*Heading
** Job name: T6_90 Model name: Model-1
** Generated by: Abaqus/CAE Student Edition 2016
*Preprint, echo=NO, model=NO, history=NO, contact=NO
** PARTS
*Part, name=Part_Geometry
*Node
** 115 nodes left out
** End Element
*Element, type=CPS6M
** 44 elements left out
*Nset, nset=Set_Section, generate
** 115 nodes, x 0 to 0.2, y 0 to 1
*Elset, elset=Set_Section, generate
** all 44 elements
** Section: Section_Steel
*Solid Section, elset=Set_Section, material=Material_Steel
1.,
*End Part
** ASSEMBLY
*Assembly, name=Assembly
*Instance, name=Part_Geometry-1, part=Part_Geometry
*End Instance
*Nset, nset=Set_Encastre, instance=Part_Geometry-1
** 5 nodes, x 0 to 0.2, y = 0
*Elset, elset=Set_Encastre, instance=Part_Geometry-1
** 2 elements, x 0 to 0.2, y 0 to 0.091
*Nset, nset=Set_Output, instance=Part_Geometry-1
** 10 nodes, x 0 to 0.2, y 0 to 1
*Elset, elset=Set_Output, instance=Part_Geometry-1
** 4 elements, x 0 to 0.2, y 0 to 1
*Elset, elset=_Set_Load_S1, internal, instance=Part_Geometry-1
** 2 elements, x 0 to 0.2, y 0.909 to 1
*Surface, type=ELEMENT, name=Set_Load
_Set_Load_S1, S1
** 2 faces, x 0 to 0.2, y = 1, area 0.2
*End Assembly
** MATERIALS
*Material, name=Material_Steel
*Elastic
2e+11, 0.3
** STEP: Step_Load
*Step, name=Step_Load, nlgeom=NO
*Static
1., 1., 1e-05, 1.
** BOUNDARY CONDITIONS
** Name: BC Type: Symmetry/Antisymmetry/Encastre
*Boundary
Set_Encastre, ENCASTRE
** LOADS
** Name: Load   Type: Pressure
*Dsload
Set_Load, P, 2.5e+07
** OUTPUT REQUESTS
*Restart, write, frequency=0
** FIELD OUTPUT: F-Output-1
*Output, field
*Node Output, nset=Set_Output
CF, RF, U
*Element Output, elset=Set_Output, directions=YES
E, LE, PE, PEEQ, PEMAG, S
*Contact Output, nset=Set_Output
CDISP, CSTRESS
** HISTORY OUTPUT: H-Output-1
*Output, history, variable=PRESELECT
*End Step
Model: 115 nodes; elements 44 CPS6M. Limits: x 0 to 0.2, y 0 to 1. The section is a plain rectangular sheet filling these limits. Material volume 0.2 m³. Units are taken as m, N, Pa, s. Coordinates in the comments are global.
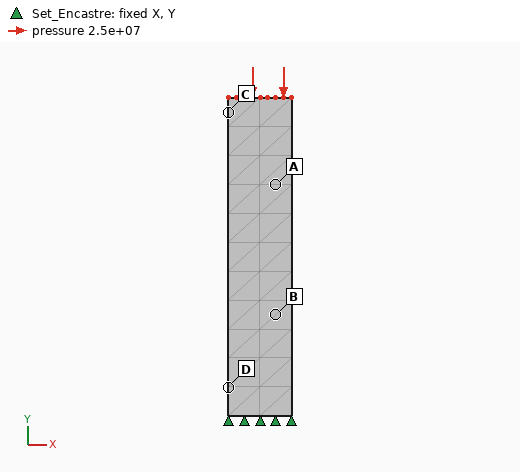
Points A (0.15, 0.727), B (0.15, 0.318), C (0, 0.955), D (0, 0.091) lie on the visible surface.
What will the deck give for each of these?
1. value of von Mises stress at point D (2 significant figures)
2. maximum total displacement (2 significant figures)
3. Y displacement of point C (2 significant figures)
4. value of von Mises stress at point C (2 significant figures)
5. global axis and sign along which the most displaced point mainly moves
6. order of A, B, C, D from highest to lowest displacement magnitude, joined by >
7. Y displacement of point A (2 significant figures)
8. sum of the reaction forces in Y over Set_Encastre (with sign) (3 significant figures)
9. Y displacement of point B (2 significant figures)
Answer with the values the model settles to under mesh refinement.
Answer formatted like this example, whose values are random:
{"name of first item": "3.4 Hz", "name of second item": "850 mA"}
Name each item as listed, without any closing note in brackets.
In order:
{"value of von Mises stress at point D": "2.4e+07 Pa", "maximum total displacement": "1.2e-04 m", "Y displacement of point C": "-1.2e-04 m", "value of von Mises stress at point C": "2.5e+07 Pa", "global axis and sign along which the most displaced point mainly moves": "-Y", "order of A, B, C, D from highest to lowest displacement magnitude, joined by >": "C > A > B > D", "Y displacement of point A": "-9.1e-05 m", "sum of the reaction forces in Y over Set_Encastre (with sign)": "5.00e+06 N", "Y displacement of point B": "-3.9e-05 m"}
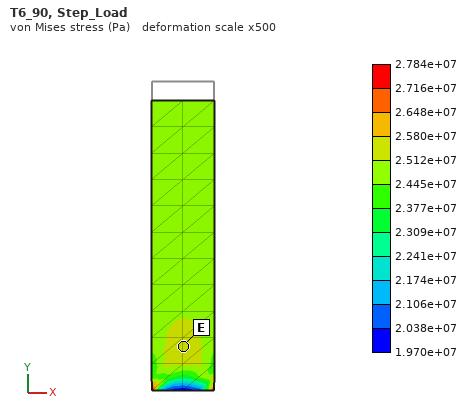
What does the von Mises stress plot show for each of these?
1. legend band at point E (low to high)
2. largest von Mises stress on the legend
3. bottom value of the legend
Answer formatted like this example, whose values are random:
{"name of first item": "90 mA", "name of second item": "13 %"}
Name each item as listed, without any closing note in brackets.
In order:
{"legend band at point E": "2.512e+07 to 2.580e+07 Pa", "largest von Mises stress on the legend": "2.784e+07 Pa", "bottom value of the legend": "1.970e+07 Pa"}
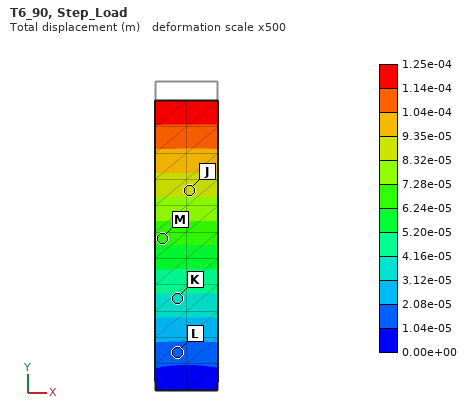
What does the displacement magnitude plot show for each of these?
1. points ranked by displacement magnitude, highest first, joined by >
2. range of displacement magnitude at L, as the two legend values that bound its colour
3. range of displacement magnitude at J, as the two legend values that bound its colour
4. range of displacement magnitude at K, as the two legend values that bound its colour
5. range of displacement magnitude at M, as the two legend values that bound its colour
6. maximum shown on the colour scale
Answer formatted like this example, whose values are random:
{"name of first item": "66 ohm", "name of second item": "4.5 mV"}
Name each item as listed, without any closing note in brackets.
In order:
{"points ranked by displacement magnitude, highest first, joined by >": "J > M > K > L", "range of displacement magnitude at L, as the two legend values that bound its colour": "1.04e-05 to 2.08e-05 m", "range of displacement magnitude at J, as the two legend values that bound its colour": "8.32e-05 to 9.35e-05 m", "range of displacement magnitude at K, as the two legend values that bound its colour": "3.12e-05 to 4.16e-05 m", "range of displacement magnitude at M, as the two legend values that bound its colour": "6.24e-05 to 7.28e-05 m", "maximum shown on the colour scale": "1.25e-04 m"}
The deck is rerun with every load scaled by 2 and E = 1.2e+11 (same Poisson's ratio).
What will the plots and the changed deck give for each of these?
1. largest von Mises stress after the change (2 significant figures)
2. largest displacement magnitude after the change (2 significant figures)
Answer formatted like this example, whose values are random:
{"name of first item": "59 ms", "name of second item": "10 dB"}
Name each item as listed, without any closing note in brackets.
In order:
{"largest von Mises stress after the change": "5.6e+07 Pa", "largest displacement magnitude after the change": "4.2e-04 m"}
